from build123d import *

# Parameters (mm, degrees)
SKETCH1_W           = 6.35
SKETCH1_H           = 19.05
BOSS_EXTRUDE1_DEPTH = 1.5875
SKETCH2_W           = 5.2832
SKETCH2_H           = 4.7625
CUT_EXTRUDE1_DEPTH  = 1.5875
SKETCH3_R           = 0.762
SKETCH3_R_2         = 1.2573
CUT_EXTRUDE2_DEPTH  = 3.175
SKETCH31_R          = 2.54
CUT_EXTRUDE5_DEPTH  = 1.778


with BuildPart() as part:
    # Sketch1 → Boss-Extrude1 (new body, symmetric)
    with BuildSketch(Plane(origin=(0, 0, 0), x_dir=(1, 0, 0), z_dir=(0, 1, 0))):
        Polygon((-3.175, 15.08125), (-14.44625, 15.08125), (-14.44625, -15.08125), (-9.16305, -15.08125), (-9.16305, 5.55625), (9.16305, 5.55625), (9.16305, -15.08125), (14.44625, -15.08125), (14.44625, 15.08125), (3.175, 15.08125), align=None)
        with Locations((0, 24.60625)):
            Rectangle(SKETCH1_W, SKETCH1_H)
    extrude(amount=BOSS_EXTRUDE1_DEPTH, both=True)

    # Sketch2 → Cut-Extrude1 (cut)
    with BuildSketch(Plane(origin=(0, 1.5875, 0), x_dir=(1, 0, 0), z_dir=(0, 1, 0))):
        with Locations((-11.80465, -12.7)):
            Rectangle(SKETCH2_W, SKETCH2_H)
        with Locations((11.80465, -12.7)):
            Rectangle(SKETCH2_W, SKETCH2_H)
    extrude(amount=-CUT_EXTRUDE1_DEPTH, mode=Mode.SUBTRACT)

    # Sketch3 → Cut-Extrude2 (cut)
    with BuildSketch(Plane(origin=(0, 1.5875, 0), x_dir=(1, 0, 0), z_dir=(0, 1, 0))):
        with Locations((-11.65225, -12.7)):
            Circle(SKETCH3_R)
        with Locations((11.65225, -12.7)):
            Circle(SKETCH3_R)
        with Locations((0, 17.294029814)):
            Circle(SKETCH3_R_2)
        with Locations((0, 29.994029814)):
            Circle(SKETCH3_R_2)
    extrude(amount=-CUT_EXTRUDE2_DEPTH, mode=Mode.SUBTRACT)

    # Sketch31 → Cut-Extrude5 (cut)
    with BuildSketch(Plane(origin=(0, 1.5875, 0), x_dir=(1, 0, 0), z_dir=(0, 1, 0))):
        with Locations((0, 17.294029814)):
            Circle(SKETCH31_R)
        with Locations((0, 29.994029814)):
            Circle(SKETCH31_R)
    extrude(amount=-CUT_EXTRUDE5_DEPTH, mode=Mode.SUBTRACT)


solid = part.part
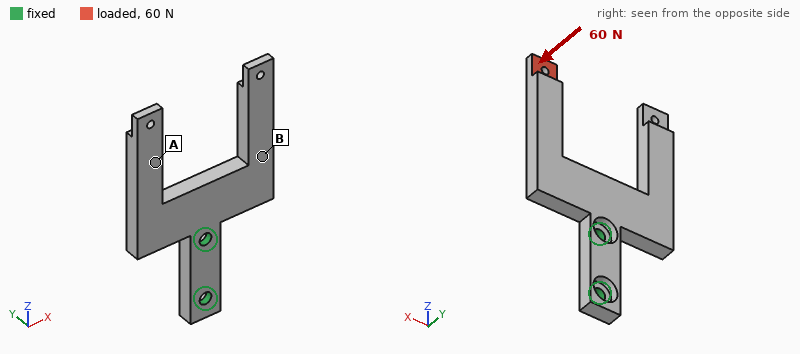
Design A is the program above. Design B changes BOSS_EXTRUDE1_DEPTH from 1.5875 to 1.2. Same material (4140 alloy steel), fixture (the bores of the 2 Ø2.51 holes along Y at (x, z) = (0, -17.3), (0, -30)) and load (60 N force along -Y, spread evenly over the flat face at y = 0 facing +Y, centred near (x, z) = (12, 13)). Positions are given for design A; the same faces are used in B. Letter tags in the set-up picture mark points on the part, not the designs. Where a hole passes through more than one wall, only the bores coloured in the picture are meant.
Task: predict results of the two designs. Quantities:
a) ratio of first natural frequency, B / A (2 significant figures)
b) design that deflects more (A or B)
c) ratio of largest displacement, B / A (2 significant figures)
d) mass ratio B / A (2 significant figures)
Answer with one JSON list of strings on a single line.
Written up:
["0.78", "B", "2.2", "0.76"]
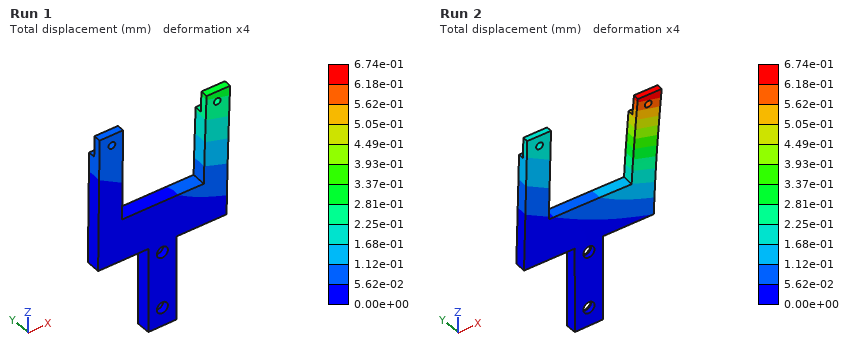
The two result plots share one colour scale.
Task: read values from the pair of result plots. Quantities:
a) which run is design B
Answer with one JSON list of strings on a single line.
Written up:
["Run 2"]
